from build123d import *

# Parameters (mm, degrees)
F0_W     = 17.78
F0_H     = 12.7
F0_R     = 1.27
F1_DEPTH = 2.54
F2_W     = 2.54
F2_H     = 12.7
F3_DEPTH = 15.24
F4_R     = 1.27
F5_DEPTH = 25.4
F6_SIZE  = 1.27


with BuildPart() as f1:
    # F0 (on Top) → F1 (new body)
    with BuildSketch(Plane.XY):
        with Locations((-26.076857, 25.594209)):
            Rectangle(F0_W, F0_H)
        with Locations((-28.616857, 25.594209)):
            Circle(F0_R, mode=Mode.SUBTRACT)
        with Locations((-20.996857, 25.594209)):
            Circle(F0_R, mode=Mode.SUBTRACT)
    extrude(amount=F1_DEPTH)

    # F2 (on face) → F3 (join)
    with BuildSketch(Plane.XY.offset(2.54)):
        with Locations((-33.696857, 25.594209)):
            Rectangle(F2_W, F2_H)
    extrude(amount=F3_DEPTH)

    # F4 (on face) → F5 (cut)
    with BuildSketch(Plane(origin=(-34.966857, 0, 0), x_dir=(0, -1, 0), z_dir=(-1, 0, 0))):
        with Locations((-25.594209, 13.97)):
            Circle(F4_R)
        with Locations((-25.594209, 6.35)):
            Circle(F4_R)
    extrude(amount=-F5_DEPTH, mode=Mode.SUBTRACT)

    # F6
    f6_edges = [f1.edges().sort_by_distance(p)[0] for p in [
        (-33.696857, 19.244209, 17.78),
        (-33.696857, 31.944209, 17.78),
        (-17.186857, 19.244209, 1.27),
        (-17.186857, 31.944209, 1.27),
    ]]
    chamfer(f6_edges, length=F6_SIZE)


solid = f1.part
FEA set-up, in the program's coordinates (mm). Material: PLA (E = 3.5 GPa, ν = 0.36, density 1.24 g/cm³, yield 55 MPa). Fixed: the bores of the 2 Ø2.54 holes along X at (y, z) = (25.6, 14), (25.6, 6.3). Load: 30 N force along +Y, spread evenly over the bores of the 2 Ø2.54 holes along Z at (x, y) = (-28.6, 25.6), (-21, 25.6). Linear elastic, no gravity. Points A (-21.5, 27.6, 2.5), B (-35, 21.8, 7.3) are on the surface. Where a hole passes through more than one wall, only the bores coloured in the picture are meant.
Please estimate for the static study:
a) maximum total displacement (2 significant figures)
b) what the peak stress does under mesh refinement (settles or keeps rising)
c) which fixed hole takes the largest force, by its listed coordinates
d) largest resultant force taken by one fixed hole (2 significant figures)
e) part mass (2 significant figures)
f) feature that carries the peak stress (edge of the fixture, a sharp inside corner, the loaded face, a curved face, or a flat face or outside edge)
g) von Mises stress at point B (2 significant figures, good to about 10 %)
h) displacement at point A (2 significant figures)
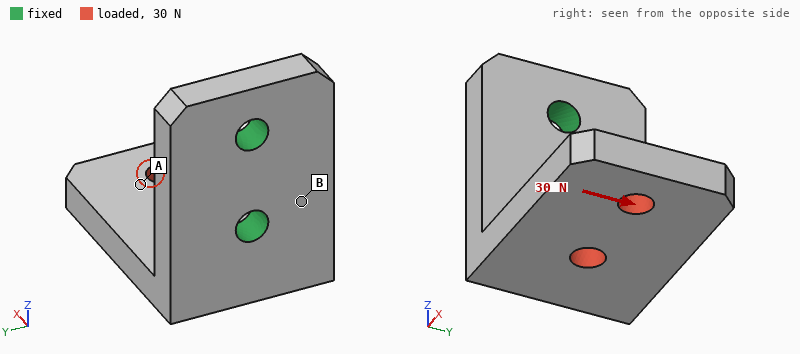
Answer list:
0.23 mm
keeps rising
(25.6, 6.3)
42 N
1.2 g
edge of the fixture
8.3 MPa
0.17 mm
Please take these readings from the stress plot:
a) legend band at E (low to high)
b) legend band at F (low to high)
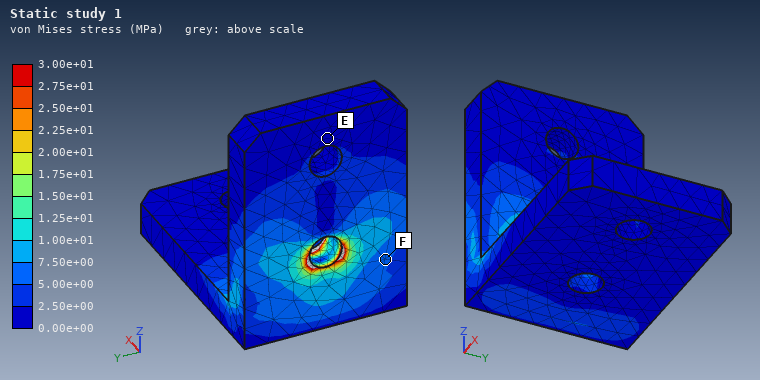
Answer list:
0.00e+00 to 2.50e+00 MPa
5.00e+00 to 7.50e+00 MPa
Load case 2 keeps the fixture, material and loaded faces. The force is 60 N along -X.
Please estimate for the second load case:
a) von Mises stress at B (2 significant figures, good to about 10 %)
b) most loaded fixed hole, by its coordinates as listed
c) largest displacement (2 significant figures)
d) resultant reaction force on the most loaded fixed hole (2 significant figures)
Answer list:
6.2 MPa
(25.6, 6.3)
0.22 mm
70 N
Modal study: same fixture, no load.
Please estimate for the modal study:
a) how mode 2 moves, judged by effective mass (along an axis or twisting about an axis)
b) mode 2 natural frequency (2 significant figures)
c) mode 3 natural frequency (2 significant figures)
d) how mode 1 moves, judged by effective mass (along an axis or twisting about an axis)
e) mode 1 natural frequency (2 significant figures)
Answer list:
along Y
2800 Hz
6200 Hz
along Z
1800 Hz
